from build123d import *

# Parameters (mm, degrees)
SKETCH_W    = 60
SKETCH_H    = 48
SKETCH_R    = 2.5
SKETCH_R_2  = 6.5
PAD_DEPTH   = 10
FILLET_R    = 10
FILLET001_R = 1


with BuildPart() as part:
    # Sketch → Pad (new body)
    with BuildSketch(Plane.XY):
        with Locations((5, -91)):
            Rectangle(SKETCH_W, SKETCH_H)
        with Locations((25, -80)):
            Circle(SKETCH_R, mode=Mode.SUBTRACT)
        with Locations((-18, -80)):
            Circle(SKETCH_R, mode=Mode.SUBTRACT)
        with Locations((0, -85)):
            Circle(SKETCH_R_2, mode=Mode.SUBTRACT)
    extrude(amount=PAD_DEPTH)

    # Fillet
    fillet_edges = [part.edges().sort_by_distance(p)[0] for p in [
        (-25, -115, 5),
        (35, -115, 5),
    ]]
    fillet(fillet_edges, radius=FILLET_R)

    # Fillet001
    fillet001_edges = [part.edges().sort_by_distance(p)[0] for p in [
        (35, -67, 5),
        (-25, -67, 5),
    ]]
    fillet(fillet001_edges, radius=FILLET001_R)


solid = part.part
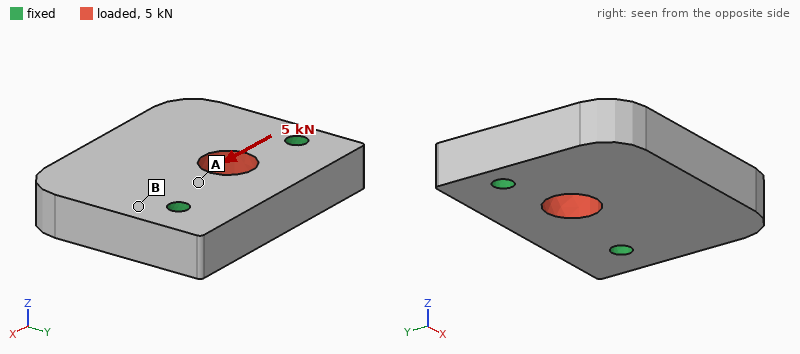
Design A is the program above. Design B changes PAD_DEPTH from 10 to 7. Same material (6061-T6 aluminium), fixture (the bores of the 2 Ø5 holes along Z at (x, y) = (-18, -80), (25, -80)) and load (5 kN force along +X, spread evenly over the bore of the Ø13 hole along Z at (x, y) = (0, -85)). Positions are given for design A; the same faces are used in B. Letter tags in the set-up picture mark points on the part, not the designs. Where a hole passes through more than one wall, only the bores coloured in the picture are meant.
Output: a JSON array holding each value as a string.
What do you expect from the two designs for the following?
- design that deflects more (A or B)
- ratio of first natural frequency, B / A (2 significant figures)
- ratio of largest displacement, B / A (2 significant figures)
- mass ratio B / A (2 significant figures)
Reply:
["B", "0.75", "1.4", "0.70"]
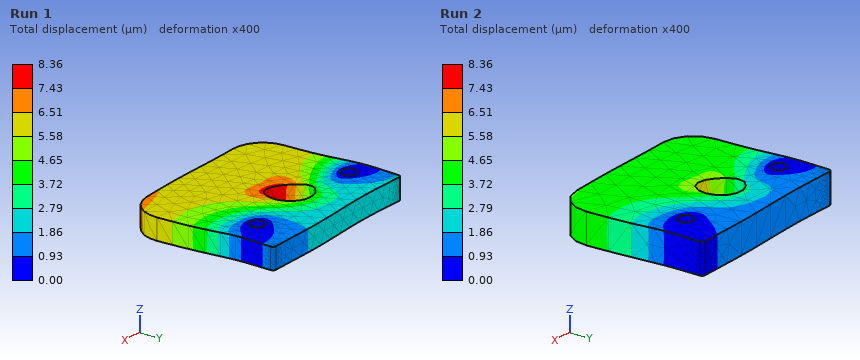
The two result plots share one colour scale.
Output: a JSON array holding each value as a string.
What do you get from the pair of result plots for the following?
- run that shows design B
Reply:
["Run 1"]
